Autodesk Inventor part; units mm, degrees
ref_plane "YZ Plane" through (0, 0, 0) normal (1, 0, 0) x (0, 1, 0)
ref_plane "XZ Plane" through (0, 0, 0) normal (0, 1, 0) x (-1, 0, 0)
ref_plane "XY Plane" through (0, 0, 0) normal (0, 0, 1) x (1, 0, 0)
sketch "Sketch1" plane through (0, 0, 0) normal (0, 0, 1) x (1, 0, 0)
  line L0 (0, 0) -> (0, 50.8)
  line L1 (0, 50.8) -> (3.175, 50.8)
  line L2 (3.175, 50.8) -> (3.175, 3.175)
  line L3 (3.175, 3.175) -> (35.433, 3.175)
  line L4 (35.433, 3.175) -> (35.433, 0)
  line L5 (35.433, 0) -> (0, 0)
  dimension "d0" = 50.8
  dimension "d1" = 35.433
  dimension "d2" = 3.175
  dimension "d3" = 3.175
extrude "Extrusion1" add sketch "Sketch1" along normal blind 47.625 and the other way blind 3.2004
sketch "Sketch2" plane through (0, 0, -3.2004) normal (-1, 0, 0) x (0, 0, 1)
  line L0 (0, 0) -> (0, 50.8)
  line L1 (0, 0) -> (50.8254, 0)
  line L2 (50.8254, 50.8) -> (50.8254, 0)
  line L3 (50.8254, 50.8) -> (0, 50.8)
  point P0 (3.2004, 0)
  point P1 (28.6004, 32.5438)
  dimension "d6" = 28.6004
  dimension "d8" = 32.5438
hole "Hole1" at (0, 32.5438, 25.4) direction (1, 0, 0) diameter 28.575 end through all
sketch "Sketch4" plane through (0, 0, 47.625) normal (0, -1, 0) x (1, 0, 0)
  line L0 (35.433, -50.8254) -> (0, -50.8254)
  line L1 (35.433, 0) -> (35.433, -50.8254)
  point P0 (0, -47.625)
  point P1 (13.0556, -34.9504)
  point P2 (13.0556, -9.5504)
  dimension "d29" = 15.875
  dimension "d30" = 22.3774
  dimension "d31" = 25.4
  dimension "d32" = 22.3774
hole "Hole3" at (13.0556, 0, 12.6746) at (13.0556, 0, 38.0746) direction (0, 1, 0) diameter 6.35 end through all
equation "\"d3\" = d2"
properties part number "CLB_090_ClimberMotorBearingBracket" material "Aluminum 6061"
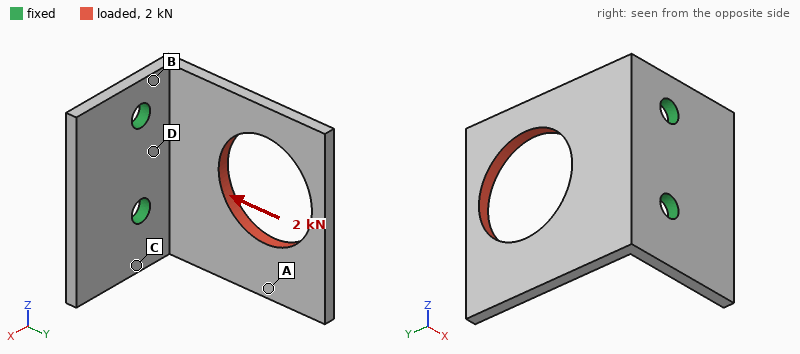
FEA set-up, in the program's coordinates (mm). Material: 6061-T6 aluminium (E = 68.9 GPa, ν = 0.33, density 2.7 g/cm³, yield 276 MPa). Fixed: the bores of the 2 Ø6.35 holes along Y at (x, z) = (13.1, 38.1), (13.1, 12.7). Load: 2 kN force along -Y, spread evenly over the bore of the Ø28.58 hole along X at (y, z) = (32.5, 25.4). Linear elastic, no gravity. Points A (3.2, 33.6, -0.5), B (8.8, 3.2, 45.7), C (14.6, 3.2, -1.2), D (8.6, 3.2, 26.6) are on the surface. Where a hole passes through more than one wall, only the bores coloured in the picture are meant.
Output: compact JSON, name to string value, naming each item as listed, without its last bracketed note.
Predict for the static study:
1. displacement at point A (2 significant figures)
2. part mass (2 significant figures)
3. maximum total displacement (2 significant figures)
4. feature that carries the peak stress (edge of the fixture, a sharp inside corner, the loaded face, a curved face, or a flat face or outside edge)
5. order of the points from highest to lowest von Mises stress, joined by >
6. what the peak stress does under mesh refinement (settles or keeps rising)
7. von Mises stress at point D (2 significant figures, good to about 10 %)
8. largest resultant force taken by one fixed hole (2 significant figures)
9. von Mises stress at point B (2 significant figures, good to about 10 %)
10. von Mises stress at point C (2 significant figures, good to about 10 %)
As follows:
{"displacement at point A": "0.34 mm", "part mass": "30 g", "maximum total displacement": "0.56 mm", "feature that carries the peak stress": "edge of the fixture", "order of the points from highest to lowest von Mises stress, joined by >": "B > D > C > A", "what the peak stress does under mesh refinement": "keeps rising", "von Mises stress at point D": "87 MPa", "largest resultant force taken by one fixed hole": "1.0 kN", "von Mises stress at point B": "130 MPa", "von Mises stress at point C": "47 MPa"}
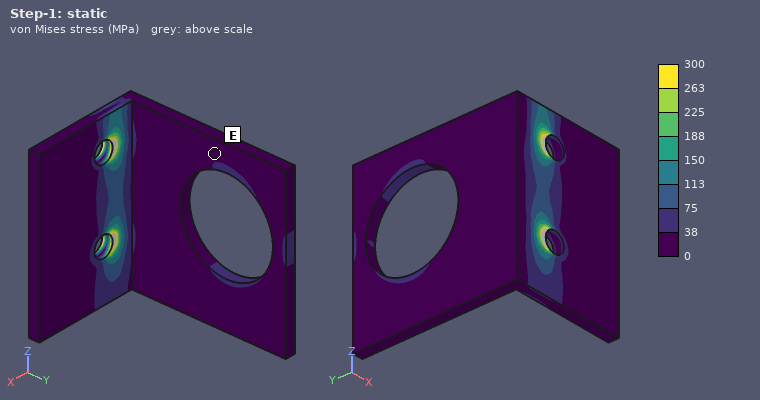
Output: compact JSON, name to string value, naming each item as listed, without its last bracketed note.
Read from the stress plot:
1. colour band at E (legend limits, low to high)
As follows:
{"colour band at E": "0 to 38 MPa"}
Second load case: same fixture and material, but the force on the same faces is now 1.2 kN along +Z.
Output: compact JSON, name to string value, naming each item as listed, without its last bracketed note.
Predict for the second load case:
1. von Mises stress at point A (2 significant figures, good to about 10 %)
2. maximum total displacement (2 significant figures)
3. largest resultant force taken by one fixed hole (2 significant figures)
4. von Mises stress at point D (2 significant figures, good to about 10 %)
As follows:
{"von Mises stress at point A": "25 MPa", "maximum total displacement": "0.42 mm", "largest resultant force taken by one fixed hole": "1.4 kN", "von Mises stress at point D": "65 MPa"}
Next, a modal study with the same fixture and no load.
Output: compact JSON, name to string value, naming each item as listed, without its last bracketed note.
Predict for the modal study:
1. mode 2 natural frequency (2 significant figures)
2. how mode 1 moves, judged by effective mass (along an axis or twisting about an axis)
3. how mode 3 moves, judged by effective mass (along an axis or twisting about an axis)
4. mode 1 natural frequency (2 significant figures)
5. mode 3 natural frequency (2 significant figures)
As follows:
{"mode 2 natural frequency": "1900 Hz", "how mode 1 moves, judged by effective mass": "along X", "how mode 3 moves, judged by effective mass": "along Z", "mode 1 natural frequency": "930 Hz", "mode 3 natural frequency": "3300 Hz"}
